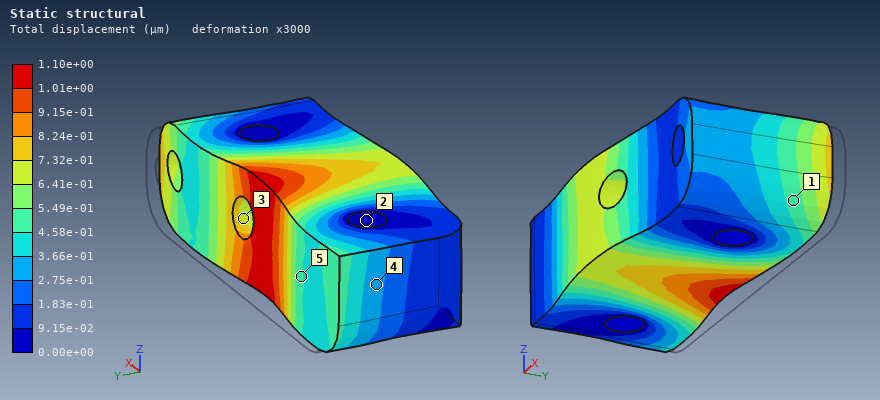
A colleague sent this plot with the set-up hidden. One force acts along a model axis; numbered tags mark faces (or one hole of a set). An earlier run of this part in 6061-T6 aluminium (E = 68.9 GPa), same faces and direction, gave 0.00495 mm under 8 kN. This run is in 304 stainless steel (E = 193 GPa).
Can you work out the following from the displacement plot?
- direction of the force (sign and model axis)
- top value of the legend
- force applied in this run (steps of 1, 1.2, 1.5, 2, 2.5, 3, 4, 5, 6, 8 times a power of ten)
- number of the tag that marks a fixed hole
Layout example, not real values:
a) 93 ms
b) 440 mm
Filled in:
a) -Y
b) 1.10e+00 µm
c) 5 kN
d) 2
